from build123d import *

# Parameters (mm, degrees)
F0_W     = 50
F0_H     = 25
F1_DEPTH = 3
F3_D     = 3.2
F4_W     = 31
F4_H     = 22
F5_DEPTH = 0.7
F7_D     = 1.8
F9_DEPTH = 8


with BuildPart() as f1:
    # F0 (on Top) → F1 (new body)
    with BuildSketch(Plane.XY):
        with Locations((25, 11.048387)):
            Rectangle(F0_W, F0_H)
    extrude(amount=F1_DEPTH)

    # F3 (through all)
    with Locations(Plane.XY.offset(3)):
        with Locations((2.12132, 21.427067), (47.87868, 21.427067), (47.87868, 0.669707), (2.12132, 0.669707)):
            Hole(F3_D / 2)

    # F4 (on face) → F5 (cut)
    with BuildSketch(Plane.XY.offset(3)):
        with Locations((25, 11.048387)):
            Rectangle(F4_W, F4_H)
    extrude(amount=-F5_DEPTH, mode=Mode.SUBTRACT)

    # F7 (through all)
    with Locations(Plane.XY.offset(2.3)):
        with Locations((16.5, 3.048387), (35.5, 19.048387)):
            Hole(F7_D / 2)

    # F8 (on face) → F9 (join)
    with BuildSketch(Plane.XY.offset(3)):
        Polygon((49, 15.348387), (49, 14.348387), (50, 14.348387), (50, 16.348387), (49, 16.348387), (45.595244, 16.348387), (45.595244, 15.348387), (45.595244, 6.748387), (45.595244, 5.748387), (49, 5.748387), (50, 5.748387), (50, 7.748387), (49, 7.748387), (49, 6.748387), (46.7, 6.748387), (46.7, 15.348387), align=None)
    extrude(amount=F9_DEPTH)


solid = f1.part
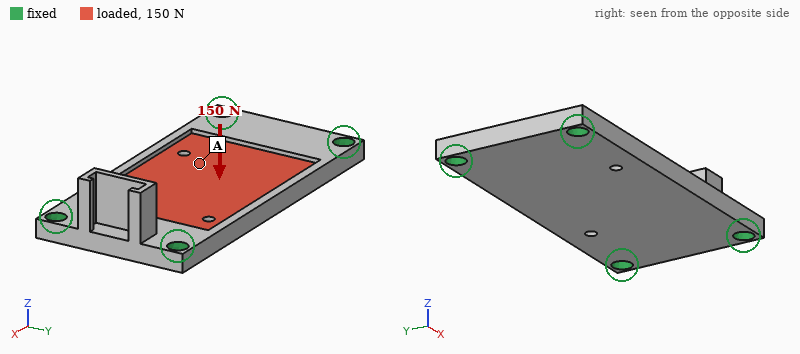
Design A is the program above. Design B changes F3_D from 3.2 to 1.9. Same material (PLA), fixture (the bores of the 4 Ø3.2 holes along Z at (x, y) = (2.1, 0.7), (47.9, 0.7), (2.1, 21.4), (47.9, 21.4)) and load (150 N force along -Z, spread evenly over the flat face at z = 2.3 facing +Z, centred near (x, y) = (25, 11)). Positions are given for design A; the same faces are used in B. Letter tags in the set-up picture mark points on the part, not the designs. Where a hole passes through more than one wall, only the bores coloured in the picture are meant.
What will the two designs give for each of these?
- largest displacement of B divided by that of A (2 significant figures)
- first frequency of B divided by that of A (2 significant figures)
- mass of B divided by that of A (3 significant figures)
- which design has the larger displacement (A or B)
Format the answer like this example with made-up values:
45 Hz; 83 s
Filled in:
1.2; 0.90; 1.02; B
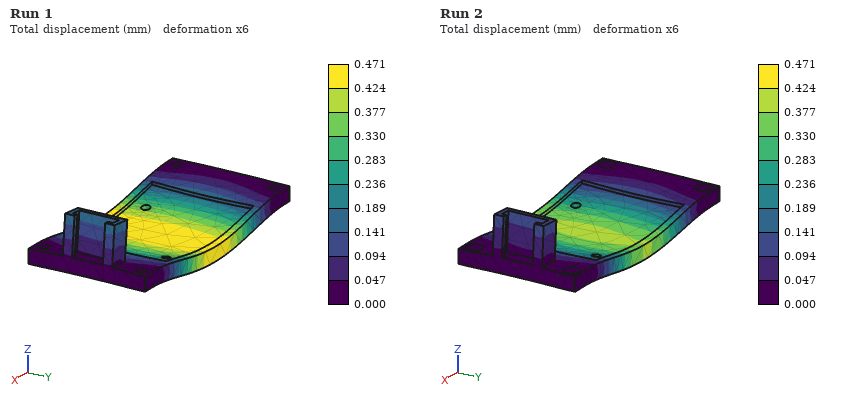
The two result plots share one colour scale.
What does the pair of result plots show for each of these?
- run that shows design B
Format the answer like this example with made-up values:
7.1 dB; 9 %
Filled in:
Run 1
